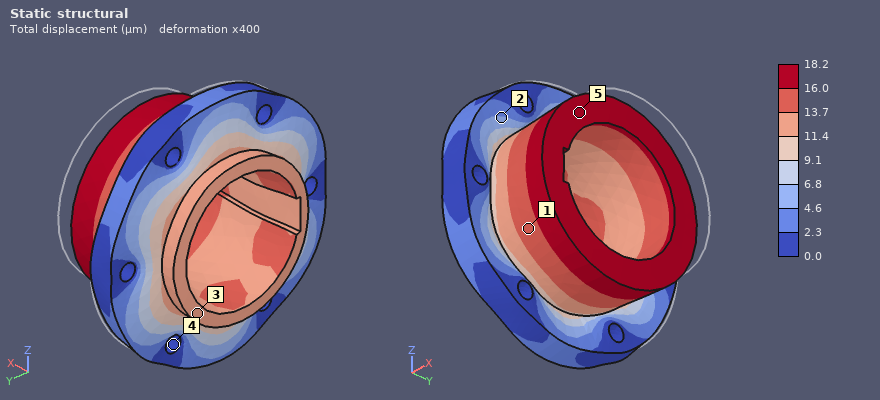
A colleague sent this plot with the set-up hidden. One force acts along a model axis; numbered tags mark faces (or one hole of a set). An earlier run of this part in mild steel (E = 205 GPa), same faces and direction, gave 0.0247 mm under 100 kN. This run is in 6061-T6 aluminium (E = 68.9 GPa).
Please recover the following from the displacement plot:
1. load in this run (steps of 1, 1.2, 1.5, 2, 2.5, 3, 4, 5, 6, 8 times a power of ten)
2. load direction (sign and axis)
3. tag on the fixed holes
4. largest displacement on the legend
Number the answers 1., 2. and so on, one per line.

1. 25 kN
2. -X
3. 4
4. 18.2 µm
